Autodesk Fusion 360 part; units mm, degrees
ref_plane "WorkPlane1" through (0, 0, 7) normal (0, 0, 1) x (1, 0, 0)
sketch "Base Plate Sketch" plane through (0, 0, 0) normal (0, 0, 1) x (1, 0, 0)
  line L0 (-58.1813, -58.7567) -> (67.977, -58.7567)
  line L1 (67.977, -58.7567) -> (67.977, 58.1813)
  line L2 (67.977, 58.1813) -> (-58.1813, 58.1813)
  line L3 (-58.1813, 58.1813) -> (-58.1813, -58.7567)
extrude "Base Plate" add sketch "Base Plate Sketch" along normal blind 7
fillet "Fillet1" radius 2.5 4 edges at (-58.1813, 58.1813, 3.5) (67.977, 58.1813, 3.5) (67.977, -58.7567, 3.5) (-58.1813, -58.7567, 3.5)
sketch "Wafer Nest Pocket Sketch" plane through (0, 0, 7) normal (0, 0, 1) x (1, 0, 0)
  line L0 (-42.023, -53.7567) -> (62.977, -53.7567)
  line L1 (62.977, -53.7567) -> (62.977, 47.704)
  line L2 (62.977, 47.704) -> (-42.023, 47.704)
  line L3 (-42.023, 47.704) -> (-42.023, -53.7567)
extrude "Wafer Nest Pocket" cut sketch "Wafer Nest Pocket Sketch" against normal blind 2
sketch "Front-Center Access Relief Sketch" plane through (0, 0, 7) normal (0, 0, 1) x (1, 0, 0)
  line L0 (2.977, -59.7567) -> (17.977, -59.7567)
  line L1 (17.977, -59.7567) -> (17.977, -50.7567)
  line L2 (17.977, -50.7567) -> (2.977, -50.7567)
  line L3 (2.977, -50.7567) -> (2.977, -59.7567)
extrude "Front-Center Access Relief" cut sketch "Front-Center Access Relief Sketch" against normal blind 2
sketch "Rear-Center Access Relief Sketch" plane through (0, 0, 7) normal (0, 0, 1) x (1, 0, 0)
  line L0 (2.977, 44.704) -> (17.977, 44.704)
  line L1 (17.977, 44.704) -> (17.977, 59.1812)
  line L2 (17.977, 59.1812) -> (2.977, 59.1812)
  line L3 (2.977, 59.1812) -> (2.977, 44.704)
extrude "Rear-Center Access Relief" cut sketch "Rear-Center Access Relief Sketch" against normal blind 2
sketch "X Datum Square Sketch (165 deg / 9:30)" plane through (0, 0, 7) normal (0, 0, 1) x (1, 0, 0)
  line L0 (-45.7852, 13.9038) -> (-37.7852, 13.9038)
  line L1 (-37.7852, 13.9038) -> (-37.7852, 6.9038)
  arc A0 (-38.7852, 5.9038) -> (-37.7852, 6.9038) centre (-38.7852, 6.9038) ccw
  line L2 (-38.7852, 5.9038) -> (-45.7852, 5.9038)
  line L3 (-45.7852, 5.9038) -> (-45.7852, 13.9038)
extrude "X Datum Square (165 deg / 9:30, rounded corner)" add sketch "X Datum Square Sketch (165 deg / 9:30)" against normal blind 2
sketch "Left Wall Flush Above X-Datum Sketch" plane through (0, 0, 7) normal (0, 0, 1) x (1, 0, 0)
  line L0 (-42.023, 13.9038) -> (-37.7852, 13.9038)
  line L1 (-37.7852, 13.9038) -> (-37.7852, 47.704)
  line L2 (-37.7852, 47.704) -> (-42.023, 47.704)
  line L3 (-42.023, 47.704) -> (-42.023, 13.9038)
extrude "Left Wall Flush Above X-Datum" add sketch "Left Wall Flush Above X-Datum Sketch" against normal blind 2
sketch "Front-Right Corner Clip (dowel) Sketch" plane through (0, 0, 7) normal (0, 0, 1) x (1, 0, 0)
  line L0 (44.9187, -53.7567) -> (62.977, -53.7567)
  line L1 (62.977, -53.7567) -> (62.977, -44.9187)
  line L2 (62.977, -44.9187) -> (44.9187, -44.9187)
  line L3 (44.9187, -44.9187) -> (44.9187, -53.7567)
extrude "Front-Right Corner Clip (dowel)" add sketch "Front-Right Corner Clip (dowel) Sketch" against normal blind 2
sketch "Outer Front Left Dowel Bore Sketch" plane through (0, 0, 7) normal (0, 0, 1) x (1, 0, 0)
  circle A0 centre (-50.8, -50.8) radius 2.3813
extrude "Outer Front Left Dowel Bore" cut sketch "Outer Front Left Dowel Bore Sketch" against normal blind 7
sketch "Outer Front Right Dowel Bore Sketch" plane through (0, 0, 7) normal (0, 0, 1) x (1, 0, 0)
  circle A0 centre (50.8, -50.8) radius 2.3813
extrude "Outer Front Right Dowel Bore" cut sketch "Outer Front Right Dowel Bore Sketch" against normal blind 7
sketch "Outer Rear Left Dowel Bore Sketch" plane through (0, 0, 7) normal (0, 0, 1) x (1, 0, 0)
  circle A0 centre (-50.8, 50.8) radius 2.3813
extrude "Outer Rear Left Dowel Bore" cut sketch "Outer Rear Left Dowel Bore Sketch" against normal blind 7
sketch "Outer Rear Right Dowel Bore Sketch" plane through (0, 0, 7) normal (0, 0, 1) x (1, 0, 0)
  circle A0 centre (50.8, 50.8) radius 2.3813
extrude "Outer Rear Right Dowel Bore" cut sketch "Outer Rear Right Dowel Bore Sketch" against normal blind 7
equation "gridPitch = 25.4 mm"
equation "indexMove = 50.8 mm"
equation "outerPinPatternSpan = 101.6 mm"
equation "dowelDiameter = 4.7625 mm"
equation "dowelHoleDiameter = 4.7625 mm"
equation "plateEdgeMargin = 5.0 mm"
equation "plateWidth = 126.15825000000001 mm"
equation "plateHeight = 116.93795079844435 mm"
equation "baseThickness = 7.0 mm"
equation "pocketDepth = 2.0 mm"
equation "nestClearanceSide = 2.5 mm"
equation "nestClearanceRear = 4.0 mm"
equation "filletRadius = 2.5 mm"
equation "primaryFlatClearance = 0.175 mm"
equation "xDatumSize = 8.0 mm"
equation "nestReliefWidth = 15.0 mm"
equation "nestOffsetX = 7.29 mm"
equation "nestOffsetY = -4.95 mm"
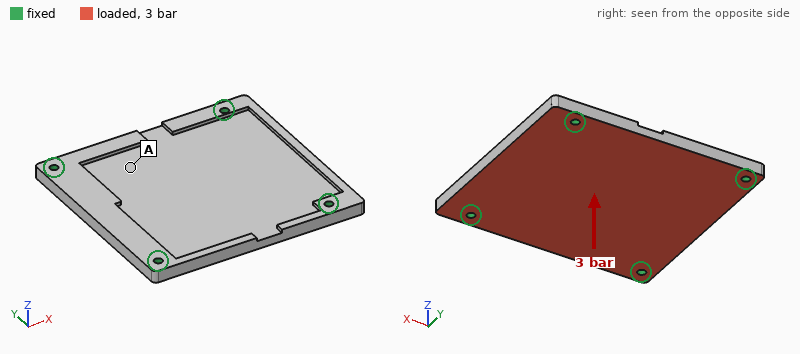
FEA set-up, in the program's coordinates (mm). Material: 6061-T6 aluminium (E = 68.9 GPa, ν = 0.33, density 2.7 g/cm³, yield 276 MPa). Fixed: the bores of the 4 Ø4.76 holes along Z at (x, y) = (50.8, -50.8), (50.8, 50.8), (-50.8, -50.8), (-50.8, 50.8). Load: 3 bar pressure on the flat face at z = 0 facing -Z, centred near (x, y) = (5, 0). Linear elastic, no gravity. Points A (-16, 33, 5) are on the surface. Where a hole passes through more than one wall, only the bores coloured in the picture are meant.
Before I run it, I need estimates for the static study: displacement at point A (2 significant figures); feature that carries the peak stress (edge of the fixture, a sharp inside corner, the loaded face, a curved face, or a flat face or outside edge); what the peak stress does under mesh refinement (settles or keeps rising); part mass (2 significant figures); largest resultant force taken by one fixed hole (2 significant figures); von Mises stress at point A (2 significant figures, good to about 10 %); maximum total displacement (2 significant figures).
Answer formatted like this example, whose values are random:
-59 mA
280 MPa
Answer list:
0.14 mm
edge of the fixture
keeps rising
220 g
1.3 kN
17 MPa
0.23 mm
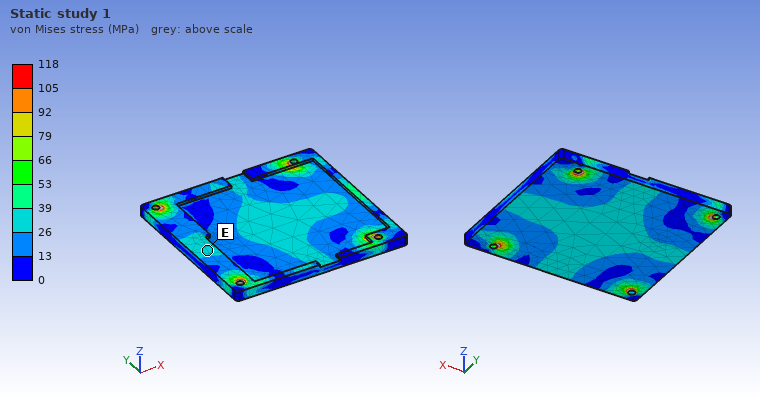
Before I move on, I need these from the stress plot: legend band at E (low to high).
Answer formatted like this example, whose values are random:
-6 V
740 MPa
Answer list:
26 to 39 MPa
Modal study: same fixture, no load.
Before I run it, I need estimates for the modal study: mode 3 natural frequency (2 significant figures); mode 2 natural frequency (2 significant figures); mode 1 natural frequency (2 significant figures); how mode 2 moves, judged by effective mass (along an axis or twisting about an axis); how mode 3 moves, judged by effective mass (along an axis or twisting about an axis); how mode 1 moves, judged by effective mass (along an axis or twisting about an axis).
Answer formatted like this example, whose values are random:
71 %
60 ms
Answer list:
3200 Hz
3000 Hz
1900 Hz
twisting about Y
twisting about X
along Z
